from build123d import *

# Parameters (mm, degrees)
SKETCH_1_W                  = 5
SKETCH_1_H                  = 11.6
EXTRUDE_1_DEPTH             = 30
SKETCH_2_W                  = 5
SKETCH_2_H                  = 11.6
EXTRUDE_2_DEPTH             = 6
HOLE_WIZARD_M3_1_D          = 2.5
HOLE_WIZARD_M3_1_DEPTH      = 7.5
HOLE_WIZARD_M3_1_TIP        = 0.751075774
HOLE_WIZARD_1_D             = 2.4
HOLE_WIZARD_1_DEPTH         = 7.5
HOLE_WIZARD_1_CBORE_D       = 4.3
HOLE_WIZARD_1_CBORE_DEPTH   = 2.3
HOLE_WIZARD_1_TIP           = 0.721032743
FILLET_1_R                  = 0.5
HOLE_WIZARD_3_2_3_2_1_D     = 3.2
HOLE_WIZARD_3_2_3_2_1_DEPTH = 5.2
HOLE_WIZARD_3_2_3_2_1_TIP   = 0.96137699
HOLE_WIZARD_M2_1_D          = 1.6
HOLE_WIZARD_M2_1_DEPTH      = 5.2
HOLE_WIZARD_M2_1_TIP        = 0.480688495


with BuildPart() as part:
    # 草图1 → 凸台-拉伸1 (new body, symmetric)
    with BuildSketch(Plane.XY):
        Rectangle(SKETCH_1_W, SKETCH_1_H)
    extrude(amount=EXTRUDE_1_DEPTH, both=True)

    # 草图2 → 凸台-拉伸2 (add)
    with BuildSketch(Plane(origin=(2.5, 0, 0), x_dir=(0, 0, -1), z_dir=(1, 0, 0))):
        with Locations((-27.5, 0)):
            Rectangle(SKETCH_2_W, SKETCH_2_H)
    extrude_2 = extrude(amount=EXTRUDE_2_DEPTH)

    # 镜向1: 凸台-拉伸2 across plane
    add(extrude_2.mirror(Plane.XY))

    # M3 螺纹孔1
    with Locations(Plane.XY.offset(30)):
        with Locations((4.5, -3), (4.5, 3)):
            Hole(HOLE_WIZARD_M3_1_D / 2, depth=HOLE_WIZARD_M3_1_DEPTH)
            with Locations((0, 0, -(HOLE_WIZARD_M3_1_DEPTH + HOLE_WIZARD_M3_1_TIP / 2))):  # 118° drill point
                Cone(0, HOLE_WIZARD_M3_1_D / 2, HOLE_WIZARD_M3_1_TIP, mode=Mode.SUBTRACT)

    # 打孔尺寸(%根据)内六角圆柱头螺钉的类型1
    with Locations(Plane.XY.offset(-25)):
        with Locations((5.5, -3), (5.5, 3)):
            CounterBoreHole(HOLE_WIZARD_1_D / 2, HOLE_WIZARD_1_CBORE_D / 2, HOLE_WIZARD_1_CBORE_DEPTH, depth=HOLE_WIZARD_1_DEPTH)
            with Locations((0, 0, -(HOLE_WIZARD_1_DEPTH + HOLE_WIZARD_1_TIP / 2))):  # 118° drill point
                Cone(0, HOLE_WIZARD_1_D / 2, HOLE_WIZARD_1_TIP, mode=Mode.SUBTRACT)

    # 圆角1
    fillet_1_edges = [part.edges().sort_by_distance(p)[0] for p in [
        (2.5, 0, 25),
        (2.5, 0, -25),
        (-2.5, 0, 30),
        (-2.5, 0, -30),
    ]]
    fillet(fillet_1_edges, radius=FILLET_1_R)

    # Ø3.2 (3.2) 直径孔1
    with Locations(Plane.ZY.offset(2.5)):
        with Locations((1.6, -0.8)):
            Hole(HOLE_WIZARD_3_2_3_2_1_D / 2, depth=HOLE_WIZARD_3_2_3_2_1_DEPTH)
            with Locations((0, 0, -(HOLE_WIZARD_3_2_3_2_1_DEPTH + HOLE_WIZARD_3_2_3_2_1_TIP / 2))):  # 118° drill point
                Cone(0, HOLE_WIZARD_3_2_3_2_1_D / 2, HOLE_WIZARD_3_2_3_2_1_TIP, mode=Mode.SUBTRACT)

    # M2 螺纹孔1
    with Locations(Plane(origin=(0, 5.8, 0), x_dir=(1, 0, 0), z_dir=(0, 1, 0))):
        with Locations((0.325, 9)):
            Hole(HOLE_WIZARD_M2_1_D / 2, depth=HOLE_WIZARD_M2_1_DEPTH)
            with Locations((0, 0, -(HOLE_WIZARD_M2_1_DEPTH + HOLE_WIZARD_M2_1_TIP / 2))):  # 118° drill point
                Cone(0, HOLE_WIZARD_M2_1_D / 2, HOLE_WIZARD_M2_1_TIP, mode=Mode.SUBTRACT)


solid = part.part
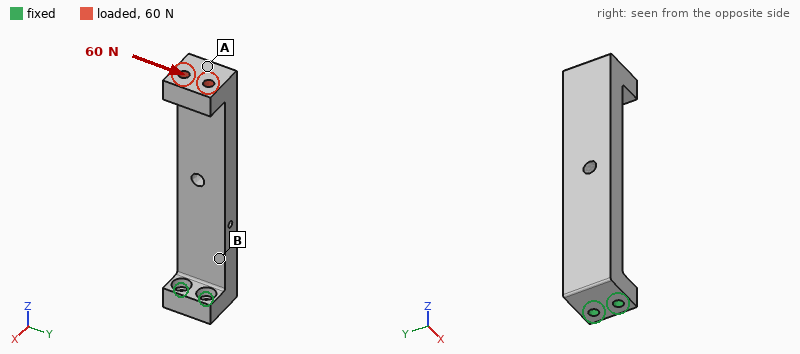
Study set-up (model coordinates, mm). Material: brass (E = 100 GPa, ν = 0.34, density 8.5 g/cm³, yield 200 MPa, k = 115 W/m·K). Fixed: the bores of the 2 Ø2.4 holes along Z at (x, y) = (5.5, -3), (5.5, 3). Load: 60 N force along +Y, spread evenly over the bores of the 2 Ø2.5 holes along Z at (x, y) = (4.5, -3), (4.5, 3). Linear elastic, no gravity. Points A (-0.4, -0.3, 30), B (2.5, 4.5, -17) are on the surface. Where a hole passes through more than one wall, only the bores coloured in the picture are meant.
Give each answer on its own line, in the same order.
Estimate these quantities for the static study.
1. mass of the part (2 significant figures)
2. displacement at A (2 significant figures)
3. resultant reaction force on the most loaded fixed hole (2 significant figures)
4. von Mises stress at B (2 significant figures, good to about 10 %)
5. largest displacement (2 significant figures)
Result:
34 g
0.11 mm
410 N
21 MPa
0.13 mm
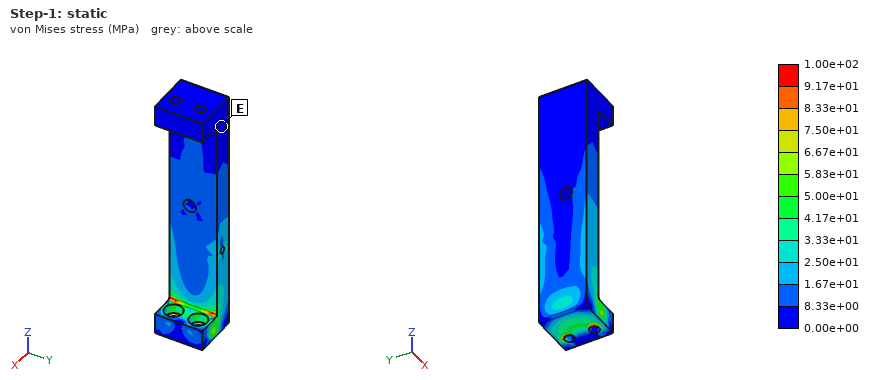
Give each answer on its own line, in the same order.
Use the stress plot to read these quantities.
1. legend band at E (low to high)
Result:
0.00e+00 to 8.33e+00 MPa
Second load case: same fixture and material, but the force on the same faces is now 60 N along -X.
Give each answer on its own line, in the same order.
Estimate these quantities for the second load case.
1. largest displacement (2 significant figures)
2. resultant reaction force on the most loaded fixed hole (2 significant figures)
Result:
0.45 mm
31 N
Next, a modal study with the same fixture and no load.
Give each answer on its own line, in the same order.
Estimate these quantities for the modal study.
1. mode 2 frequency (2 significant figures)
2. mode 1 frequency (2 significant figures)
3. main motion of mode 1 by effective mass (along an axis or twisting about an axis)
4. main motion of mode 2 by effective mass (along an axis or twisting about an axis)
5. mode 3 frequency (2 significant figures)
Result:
1100 Hz
570 Hz
along X
along Y
3600 Hz
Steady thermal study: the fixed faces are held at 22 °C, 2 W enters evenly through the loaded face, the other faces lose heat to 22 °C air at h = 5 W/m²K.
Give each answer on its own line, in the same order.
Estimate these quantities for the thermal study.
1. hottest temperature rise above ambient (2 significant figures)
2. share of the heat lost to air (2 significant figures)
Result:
19 K
5.9 %
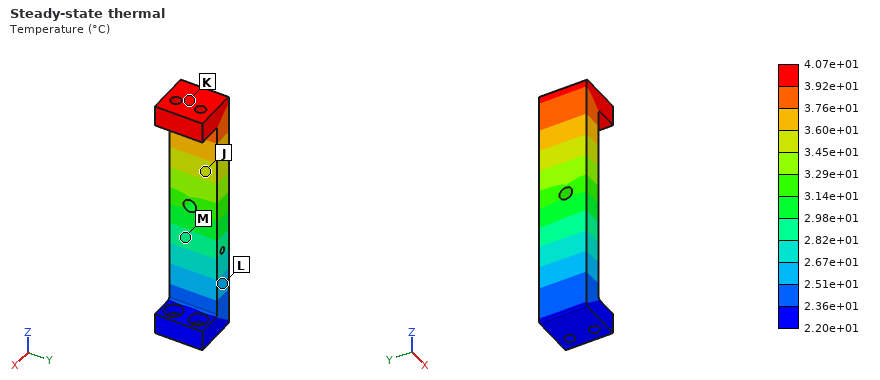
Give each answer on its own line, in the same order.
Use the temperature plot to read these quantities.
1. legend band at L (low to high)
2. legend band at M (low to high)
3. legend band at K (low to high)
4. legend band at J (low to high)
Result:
2.51e+01 to 2.67e+01 °C
2.82e+01 to 2.98e+01 °C
3.92e+01 to 4.07e+01 °C
3.45e+01 to 3.60e+01 °C
